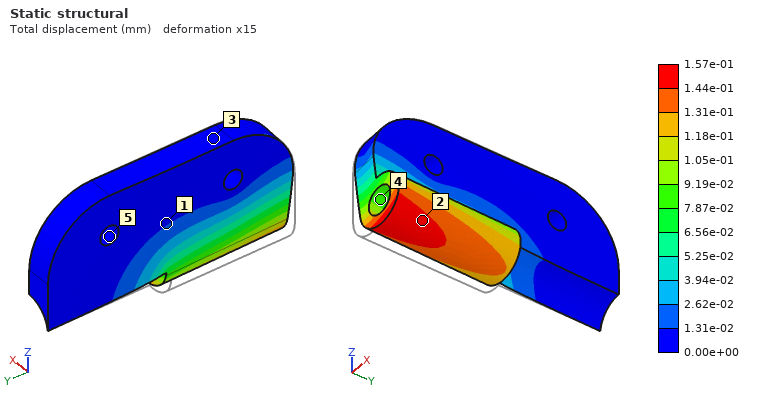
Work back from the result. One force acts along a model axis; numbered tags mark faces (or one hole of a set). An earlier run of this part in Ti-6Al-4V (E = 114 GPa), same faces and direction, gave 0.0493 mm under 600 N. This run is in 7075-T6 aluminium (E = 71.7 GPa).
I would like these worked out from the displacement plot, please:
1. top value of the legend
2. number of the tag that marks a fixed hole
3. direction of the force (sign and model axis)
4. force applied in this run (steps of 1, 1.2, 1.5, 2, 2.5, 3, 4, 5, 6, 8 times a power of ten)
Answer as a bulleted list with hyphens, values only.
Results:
- 1.57e-01 mm
- 5
- +X
- 1.2 kN
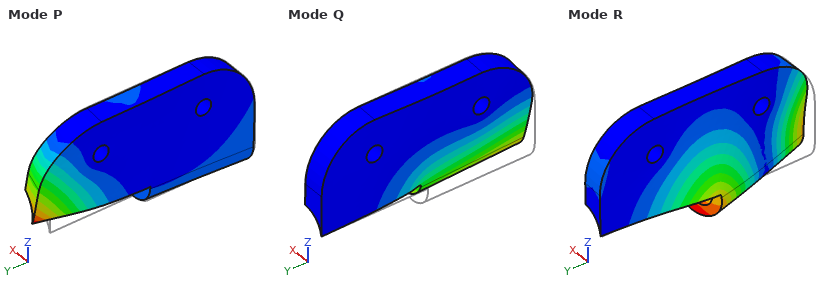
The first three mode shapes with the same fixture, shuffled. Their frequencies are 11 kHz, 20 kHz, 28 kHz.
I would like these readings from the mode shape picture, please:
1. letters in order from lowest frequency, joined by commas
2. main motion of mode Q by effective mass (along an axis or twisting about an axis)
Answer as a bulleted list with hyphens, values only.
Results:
- Q, R, P
- along X
